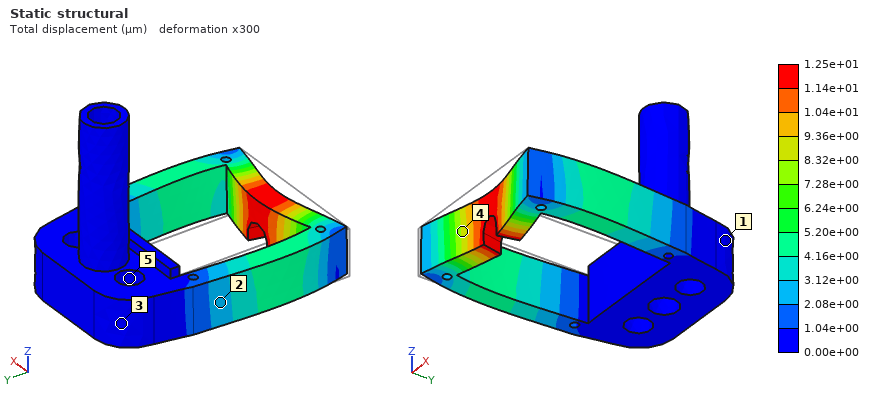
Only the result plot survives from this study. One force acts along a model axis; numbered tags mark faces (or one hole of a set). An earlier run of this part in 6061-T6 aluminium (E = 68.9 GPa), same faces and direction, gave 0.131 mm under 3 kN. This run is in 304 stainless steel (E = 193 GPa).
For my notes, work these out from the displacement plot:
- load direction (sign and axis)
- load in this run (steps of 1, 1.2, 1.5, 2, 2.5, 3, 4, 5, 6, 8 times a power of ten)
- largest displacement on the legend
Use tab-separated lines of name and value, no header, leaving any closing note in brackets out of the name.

load direction	+Y
load in this run	800 N
largest displacement on the legend	1.25e+01 µm
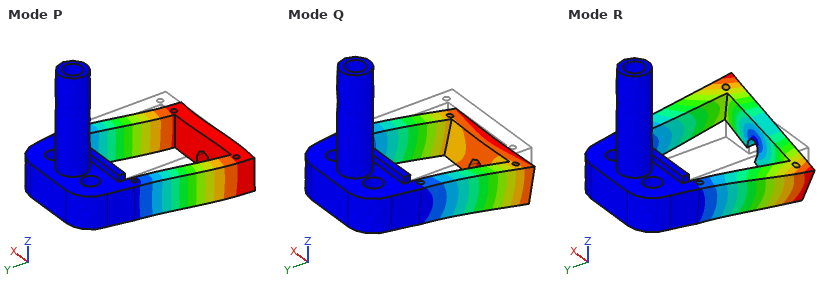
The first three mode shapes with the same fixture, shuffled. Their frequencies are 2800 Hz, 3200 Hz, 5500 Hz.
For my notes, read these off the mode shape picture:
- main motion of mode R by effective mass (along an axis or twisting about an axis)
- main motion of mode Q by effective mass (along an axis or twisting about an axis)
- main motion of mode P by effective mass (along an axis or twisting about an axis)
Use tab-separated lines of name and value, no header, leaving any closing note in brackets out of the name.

main motion of mode R by effective mass	twisting about Y
main motion of mode Q by effective mass	along Z
main motion of mode P by effective mass	along X
